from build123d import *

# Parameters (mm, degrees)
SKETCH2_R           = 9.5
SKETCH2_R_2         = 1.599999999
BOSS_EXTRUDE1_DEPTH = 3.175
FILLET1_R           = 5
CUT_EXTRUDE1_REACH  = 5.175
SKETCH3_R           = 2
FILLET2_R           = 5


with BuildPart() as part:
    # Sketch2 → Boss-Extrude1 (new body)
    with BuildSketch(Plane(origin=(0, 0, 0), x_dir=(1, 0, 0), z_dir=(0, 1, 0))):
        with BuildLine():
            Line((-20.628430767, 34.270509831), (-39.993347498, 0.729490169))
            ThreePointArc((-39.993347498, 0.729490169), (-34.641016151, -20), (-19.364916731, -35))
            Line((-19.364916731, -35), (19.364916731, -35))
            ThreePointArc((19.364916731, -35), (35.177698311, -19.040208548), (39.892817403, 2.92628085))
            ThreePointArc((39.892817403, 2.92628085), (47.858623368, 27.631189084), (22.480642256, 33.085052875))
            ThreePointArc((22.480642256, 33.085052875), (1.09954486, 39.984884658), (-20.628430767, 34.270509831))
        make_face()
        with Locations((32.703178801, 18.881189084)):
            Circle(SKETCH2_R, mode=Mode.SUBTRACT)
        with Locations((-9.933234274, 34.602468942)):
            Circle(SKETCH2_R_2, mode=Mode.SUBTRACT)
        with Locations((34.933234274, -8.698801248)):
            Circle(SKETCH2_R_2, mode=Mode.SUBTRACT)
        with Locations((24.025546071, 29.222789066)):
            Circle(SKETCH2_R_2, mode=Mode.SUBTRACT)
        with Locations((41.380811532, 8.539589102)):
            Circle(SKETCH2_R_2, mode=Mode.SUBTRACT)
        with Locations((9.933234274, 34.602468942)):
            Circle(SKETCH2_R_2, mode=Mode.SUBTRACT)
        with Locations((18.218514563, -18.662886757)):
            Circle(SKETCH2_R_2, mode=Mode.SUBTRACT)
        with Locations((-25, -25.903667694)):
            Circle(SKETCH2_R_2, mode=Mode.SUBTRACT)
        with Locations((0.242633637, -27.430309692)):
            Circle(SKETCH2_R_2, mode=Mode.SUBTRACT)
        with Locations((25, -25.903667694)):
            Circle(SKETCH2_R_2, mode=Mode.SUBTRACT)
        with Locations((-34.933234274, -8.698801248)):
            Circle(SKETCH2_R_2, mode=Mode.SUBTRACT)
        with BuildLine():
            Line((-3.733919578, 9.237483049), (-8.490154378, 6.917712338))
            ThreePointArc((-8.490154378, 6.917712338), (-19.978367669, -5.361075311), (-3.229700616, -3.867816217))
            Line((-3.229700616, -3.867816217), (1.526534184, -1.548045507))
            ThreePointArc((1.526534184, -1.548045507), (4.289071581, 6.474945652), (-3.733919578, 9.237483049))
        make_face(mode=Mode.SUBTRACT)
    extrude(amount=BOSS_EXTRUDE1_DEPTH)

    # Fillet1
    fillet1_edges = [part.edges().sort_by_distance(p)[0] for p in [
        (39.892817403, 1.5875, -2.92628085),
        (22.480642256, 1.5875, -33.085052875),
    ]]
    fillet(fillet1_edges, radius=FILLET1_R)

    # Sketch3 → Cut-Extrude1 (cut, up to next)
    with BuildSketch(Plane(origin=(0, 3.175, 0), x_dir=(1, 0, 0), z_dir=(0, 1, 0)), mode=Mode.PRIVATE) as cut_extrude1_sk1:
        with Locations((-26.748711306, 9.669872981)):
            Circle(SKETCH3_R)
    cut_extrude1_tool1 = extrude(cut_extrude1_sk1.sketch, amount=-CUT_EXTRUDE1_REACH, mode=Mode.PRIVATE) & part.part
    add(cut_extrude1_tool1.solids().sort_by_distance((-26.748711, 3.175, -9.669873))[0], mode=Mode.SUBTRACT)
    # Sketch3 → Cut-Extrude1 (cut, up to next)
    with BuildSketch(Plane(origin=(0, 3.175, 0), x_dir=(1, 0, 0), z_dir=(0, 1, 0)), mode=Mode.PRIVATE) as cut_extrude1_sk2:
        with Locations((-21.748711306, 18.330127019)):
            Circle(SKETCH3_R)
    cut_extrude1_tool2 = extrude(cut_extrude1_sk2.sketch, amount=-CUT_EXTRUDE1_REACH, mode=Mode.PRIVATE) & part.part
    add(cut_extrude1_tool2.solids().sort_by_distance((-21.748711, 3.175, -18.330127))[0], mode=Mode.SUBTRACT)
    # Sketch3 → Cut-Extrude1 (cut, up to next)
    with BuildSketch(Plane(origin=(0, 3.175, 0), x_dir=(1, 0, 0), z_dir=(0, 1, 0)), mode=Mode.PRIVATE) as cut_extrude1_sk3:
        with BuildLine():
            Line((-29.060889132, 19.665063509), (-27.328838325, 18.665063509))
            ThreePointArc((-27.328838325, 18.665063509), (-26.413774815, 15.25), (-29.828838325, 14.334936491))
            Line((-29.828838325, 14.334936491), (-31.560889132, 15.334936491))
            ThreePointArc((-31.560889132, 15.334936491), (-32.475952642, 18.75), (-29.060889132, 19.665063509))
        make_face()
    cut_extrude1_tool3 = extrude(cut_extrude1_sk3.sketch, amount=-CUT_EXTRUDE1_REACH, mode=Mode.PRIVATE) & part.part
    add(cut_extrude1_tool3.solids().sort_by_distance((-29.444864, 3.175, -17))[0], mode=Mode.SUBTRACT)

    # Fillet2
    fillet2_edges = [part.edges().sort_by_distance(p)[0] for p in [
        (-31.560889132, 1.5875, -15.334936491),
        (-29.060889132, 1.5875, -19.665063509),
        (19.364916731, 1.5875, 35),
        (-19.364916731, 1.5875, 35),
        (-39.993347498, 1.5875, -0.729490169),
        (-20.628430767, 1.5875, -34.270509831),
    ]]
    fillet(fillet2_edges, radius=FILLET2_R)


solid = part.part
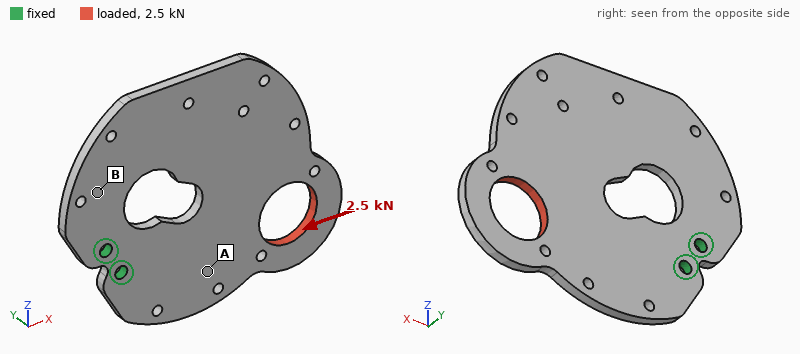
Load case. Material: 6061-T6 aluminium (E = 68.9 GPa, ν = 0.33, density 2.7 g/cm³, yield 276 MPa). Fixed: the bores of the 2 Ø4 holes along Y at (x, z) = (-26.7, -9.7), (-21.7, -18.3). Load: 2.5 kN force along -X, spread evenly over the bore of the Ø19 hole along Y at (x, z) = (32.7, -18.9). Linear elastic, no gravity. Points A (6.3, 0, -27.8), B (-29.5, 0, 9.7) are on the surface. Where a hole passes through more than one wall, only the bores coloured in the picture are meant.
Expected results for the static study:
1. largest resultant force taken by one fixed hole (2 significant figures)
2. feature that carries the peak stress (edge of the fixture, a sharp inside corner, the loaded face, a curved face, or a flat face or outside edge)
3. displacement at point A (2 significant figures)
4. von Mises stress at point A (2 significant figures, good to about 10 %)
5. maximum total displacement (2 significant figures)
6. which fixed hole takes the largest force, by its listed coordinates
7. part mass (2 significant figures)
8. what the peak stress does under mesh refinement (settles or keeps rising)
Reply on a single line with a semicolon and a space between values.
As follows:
2.3 kN; edge of the fixture; 32 µm; 25 MPa; 70 µm; (-21.7, -18.3); 38 g; keeps rising
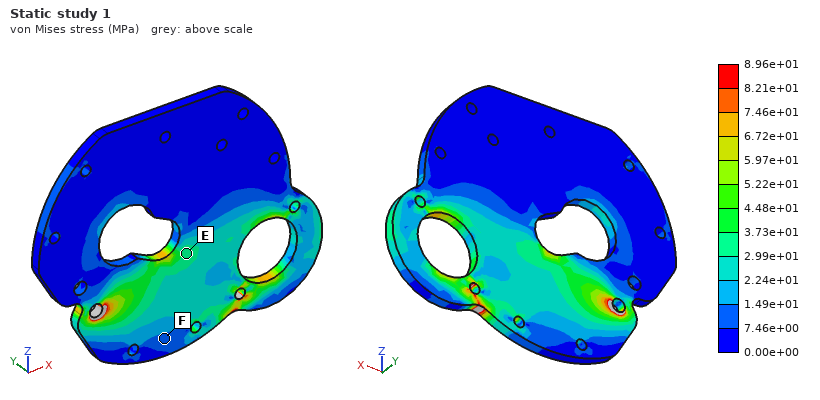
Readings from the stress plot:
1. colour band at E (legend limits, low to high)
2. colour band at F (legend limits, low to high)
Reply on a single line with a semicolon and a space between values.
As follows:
2.99e+01 to 3.73e+01 MPa; 7.46e+00 to 1.49e+01 MPa
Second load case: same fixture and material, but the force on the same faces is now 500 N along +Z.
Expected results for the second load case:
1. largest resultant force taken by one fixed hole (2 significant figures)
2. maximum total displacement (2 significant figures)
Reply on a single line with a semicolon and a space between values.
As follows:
1.9 kN; 0.16 mm
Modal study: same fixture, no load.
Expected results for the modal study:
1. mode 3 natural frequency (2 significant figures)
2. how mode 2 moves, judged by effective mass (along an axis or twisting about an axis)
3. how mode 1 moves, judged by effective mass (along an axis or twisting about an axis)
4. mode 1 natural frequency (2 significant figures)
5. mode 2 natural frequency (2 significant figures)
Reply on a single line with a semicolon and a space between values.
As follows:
2000 Hz; twisting about X; along Y; 480 Hz; 880 Hz
